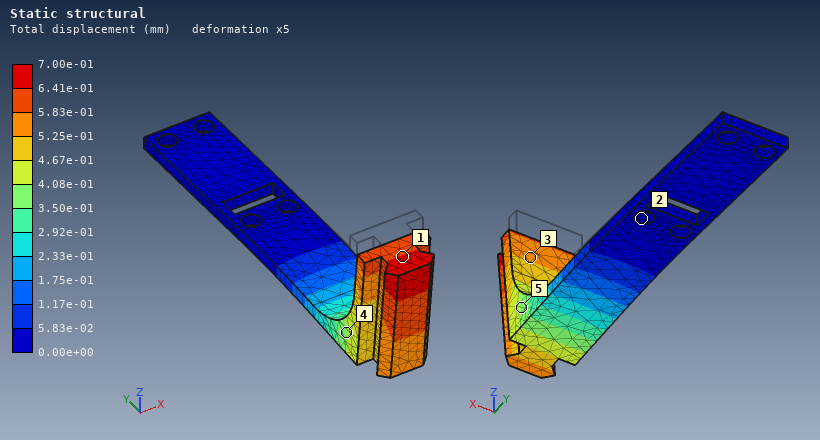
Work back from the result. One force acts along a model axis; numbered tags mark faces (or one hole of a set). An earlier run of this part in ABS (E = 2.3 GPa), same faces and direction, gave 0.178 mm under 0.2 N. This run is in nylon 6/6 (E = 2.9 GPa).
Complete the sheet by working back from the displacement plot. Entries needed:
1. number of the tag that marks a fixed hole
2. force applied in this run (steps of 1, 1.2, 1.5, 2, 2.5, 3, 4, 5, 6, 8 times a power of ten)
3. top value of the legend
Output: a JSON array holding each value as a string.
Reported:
["2", "1 N", "7.00e-01 mm"]
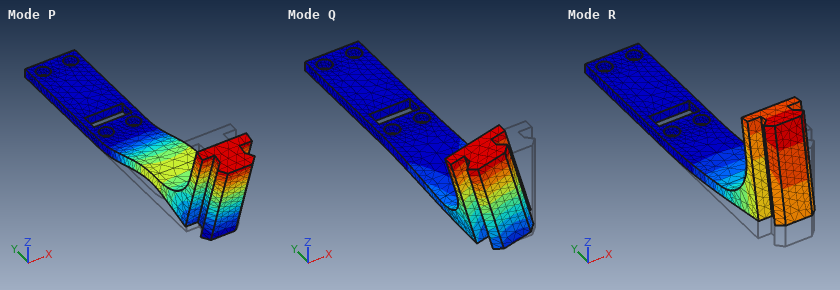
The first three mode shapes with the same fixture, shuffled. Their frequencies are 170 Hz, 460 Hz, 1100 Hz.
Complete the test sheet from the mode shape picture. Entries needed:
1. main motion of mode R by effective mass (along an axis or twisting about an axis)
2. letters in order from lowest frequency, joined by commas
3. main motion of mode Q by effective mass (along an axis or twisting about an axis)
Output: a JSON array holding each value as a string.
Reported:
["along Z", "R, Q, P", "along X"]
